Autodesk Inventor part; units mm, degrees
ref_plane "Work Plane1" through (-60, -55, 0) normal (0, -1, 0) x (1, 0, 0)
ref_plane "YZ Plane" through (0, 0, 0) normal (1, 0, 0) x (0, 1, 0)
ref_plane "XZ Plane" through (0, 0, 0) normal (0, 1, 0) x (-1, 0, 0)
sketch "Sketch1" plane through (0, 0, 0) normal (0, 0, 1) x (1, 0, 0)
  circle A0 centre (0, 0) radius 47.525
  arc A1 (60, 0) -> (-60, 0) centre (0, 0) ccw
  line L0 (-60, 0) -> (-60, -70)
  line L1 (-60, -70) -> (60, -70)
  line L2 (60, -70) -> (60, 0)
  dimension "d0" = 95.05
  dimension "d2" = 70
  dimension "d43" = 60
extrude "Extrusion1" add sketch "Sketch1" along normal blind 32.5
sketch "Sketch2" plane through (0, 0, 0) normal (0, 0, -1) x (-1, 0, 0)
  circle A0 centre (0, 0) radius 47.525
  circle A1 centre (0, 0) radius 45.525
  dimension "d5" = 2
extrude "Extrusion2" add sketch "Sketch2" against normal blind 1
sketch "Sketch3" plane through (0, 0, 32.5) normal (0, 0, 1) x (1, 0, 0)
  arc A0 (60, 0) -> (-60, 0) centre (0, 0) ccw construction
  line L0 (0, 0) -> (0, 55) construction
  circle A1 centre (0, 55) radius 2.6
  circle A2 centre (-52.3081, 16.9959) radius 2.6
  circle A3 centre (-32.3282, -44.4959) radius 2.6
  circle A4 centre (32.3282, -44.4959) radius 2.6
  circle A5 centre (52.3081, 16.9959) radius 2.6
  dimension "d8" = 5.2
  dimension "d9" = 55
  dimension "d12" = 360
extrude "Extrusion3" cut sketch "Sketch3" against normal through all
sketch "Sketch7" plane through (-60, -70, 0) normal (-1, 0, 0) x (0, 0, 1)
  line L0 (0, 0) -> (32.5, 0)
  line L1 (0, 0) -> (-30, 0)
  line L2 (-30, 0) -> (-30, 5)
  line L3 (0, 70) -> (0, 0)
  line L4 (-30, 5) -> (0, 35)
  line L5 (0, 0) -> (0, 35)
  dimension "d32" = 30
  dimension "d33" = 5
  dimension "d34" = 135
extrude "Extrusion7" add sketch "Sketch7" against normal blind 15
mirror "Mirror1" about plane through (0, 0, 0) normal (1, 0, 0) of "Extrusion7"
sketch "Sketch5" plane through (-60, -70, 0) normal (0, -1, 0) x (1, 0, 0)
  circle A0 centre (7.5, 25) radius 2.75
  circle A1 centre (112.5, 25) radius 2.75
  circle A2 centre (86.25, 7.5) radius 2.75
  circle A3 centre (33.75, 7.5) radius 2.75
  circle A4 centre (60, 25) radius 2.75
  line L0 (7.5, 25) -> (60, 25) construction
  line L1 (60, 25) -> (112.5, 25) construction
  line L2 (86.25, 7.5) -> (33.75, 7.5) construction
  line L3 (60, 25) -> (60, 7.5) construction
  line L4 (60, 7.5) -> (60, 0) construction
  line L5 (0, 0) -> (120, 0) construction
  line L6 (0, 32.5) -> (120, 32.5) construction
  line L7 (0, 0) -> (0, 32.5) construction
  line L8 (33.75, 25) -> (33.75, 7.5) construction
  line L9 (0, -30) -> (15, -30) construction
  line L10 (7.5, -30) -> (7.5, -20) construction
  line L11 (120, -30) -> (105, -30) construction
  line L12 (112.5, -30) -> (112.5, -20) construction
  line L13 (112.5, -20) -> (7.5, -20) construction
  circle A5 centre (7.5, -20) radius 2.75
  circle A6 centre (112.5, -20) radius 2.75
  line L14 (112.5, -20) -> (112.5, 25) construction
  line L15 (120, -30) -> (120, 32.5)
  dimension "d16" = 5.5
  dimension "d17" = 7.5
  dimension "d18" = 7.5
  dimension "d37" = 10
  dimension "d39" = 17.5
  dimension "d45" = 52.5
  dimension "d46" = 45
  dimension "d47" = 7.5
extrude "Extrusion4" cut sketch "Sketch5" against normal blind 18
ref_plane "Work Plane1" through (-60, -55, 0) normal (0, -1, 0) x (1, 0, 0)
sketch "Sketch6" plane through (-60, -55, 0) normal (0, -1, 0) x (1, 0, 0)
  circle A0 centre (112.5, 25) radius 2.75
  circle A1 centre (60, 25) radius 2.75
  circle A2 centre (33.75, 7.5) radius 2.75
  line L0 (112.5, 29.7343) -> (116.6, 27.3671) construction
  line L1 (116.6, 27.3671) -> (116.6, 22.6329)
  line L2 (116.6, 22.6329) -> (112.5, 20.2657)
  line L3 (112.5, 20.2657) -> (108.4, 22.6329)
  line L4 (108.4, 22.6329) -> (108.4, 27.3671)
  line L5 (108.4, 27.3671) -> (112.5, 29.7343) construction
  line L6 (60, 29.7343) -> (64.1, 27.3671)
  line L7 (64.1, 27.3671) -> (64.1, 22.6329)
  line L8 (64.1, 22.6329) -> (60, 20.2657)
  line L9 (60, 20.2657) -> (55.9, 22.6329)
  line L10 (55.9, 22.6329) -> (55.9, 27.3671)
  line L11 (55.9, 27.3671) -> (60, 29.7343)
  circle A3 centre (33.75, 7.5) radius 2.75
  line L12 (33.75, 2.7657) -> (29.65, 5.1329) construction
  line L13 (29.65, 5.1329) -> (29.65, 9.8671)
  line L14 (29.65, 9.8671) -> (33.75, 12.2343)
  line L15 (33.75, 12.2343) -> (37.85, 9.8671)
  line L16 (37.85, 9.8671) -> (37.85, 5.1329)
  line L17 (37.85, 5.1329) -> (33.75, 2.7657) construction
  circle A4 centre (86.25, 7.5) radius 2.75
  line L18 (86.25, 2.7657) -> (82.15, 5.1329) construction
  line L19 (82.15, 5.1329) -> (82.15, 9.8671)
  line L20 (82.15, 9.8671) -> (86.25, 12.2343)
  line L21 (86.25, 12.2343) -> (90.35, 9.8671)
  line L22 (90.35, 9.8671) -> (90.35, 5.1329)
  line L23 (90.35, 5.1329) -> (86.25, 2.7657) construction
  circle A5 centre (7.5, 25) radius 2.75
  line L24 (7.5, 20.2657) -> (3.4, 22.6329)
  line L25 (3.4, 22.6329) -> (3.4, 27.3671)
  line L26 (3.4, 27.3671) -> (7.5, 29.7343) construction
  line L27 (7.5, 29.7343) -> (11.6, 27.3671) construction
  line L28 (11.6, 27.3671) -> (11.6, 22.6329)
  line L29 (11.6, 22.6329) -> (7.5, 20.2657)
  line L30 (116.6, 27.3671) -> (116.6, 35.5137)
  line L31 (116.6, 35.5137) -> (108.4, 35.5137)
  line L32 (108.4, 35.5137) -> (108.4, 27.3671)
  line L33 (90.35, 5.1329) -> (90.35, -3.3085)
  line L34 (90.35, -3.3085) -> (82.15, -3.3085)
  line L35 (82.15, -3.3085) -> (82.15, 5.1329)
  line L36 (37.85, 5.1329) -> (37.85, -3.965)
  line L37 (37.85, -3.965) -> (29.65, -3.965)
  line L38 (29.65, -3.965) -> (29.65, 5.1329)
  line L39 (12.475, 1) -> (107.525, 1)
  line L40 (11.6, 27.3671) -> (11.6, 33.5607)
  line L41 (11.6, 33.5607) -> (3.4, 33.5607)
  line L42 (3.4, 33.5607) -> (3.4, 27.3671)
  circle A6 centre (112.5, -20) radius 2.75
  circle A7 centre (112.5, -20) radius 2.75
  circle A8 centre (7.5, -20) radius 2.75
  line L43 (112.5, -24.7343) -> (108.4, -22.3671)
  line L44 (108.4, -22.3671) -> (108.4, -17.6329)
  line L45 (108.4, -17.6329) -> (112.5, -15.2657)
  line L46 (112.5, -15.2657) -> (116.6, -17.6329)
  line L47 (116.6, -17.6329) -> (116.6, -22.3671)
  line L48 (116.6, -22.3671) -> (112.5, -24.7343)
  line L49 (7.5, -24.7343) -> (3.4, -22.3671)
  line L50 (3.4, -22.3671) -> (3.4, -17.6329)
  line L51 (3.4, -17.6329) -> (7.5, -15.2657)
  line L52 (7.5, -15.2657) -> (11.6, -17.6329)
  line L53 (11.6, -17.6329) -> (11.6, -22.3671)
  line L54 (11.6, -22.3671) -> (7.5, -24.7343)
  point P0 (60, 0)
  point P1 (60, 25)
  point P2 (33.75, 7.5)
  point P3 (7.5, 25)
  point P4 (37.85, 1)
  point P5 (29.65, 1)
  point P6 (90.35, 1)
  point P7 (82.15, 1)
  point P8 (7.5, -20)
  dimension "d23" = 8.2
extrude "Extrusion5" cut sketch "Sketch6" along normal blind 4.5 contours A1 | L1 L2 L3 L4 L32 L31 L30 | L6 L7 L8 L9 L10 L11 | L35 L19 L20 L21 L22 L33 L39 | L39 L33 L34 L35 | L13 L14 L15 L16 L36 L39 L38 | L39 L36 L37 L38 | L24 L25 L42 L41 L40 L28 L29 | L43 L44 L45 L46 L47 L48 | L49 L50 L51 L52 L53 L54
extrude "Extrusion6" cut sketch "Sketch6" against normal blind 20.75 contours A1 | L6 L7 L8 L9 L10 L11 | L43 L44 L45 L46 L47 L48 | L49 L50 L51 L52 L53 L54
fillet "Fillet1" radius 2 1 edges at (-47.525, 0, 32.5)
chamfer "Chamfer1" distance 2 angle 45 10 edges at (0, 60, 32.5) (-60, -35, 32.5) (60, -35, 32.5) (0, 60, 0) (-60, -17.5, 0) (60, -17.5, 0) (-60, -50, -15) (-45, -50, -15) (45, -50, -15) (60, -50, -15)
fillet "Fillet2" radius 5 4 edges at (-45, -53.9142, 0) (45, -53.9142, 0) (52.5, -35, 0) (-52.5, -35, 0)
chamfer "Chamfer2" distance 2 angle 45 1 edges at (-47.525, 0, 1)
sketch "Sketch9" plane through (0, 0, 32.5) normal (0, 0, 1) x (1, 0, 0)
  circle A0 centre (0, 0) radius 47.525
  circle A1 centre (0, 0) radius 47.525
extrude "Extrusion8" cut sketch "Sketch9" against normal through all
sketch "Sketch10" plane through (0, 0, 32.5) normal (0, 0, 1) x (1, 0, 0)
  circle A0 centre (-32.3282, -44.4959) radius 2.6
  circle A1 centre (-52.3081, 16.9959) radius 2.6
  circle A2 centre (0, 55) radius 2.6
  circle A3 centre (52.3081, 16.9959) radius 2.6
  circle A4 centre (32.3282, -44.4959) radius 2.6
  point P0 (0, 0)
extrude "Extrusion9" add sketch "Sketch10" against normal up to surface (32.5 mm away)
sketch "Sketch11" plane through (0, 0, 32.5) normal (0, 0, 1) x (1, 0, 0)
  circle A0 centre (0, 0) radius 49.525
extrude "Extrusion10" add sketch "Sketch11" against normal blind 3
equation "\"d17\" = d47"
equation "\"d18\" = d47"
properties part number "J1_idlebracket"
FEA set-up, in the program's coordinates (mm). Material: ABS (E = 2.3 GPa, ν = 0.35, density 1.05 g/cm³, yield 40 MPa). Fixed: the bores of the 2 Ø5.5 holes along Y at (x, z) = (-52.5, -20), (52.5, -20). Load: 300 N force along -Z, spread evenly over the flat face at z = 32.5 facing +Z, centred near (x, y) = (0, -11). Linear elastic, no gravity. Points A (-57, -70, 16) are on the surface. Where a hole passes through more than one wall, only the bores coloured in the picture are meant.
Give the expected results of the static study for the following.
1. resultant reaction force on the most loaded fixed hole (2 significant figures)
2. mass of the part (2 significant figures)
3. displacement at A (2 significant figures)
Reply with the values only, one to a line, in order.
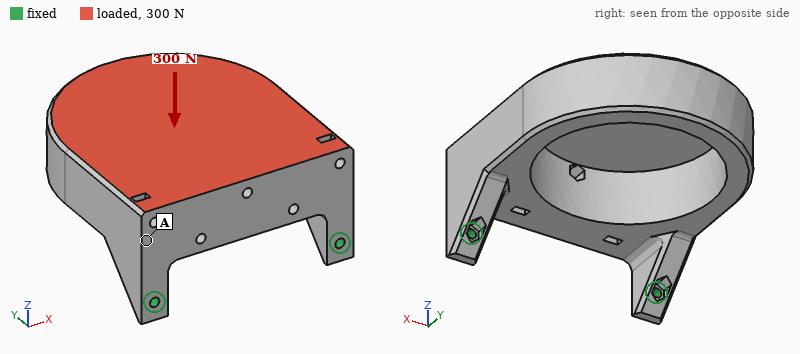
150 N
270 g
0.50 mm
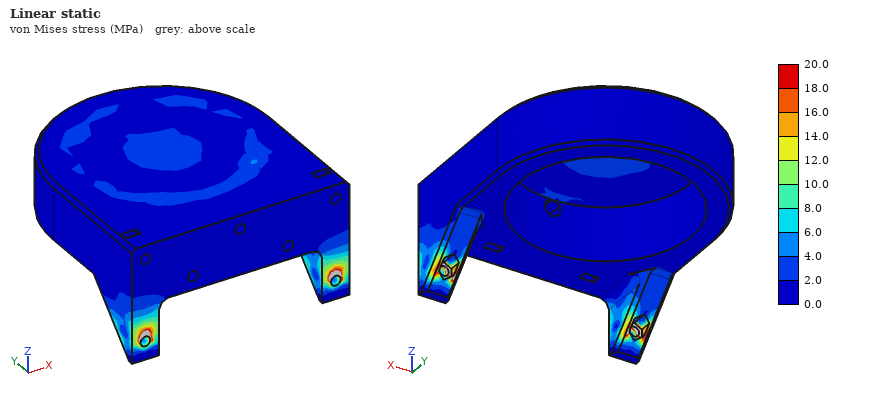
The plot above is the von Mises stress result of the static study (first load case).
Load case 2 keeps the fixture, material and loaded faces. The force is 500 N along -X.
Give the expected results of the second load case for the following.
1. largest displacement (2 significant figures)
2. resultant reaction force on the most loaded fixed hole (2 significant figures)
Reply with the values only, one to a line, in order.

0.39 mm
400 N
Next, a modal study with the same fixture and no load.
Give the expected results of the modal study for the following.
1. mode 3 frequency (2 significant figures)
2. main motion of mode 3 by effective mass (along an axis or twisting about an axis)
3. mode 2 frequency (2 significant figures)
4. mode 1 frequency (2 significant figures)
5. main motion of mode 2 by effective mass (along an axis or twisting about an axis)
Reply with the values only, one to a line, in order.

830 Hz
along Y
390 Hz
140 Hz
along X
